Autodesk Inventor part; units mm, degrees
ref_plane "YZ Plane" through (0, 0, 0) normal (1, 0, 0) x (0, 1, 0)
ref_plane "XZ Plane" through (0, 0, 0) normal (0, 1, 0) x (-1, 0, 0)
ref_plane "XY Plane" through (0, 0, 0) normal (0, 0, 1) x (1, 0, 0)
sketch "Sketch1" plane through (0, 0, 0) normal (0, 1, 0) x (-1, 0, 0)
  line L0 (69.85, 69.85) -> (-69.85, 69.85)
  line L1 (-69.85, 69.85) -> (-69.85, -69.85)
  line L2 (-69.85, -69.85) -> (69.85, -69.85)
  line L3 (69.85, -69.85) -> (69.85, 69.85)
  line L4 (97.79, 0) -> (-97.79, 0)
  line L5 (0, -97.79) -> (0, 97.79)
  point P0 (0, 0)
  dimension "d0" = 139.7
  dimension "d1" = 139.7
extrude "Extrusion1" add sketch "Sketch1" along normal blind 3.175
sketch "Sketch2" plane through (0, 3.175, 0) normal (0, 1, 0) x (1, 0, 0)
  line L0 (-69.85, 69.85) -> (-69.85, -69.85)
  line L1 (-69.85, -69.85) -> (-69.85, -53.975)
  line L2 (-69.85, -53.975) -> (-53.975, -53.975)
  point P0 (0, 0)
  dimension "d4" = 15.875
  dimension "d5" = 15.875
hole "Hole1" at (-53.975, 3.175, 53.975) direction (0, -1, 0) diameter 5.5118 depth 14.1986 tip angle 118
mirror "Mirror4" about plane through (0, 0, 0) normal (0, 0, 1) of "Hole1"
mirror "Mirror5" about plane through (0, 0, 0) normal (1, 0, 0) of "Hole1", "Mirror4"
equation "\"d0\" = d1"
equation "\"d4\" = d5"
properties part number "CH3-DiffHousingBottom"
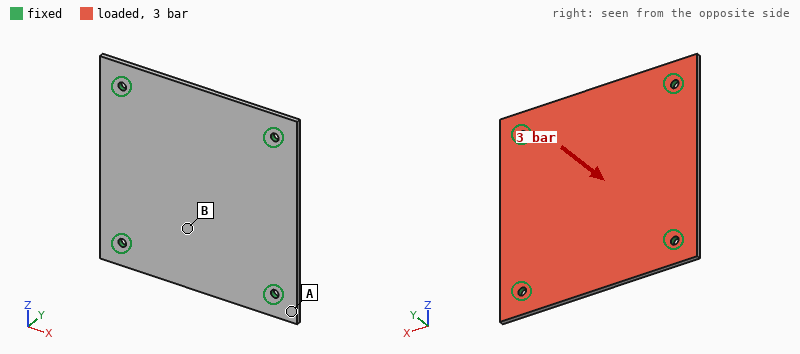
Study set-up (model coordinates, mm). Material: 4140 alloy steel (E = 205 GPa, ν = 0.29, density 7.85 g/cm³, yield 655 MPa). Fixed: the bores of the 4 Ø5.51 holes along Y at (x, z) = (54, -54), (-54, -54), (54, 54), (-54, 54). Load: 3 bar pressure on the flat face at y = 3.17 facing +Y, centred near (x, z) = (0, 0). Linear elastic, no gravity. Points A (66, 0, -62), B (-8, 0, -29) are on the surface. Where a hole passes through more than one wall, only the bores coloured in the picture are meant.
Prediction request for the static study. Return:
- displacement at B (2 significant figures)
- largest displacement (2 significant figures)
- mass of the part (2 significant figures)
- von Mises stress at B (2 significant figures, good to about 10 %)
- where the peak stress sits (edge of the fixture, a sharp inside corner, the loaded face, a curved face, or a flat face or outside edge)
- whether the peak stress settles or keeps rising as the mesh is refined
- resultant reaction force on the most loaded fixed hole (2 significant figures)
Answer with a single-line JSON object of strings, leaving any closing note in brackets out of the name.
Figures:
{"displacement at B": "0.39 mm", "largest displacement": "0.49 mm", "mass of the part": "480 g", "von Mises stress at B": "91 MPa", "where the peak stress sits": "edge of the fixture", "whether the peak stress settles or keeps rising as the mesh is refined": "keeps rising", "resultant reaction force on the most loaded fixed hole": "1.5 kN"}
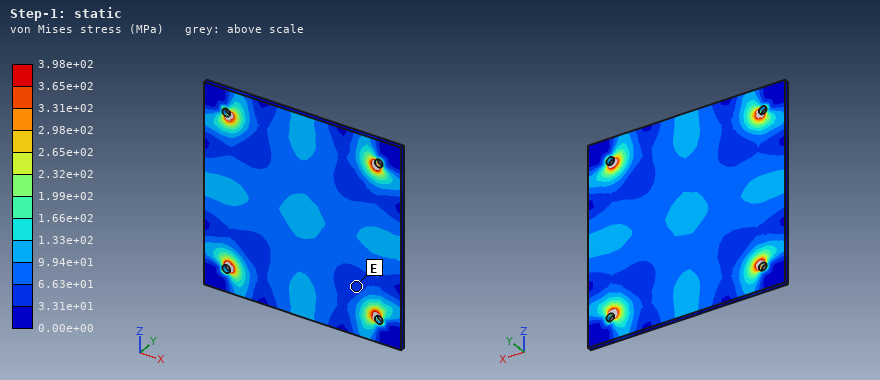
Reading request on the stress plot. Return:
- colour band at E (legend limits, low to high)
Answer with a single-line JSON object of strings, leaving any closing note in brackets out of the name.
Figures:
{"colour band at E": "3.31e+01 to 6.63e+01 MPa"}
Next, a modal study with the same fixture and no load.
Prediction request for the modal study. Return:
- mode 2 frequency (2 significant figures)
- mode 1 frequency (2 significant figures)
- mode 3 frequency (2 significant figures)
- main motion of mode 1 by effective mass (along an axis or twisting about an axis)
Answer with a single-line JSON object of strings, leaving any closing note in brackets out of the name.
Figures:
{"mode 2 frequency": "1600 Hz", "mode 1 frequency": "970 Hz", "mode 3 frequency": "1600 Hz", "main motion of mode 1 by effective mass": "along Y"}
